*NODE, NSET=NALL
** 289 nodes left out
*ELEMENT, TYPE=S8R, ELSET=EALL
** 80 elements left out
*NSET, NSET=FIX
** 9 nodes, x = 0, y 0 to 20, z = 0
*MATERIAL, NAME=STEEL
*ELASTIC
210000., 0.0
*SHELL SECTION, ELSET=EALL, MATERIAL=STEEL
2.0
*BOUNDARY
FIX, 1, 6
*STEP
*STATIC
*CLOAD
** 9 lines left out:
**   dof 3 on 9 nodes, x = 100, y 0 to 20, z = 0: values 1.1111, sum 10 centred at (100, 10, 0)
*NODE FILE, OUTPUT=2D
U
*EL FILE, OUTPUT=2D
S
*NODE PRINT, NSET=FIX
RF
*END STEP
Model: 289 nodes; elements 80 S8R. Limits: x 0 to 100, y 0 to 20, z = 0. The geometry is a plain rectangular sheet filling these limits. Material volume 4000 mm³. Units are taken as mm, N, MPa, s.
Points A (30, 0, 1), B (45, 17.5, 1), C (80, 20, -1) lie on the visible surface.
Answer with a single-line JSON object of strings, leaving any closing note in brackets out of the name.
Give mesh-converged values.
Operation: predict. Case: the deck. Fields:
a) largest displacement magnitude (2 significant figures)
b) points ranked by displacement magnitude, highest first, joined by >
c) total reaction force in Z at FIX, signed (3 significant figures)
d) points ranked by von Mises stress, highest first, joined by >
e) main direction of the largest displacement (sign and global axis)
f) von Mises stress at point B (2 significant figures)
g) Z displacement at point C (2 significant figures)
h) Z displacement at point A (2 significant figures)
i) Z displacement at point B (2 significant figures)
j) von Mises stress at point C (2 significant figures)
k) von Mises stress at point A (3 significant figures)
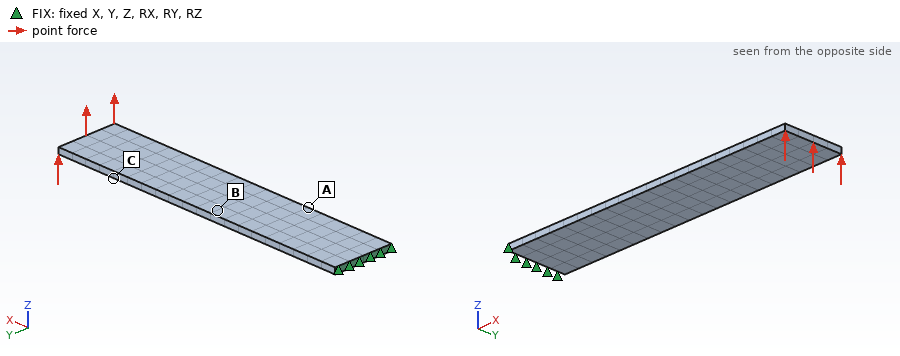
{"largest displacement magnitude": "1.2 mm", "points ranked by displacement magnitude, highest first, joined by >": "C > B > A", "total reaction force in Z at FIX, signed": "-10.0 N", "points ranked by von Mises stress, highest first, joined by >": "A > B > C", "main direction of the largest displacement": "+Z", "von Mises stress at point B": "41 MPa", "Z displacement at point C": "0.84 mm", "Z displacement at point A": "0.14 mm", "Z displacement at point B": "0.31 mm", "von Mises stress at point C": "15 MPa", "von Mises stress at point A": "52.5 MPa"}
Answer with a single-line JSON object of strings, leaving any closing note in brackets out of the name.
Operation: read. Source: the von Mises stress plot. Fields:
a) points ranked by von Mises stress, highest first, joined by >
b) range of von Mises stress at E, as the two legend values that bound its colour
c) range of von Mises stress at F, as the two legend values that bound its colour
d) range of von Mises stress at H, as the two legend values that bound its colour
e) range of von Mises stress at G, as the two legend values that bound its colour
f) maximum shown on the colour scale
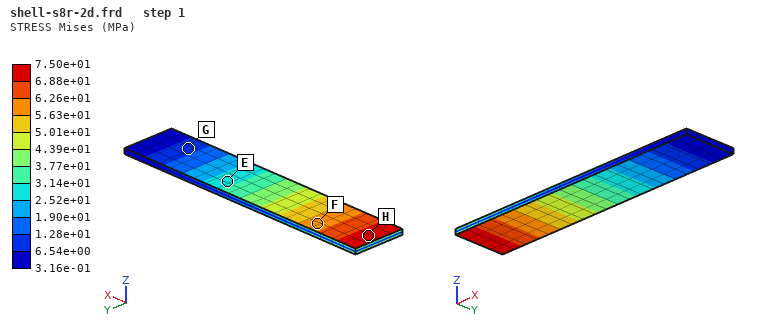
{"points ranked by von Mises stress, highest first, joined by >": "H > F > E > G", "range of von Mises stress at E, as the two legend values that bound its colour": "2.52e+01 to 3.14e+01 MPa", "range of von Mises stress at F, as the two legend values that bound its colour": "5.63e+01 to 6.26e+01 MPa", "range of von Mises stress at H, as the two legend values that bound its colour": "6.88e+01 to 7.50e+01 MPa", "range of von Mises stress at G, as the two legend values that bound its colour": "6.54e+00 to 1.28e+01 MPa", "maximum shown on the colour scale": "7.50e+01 MPa"}
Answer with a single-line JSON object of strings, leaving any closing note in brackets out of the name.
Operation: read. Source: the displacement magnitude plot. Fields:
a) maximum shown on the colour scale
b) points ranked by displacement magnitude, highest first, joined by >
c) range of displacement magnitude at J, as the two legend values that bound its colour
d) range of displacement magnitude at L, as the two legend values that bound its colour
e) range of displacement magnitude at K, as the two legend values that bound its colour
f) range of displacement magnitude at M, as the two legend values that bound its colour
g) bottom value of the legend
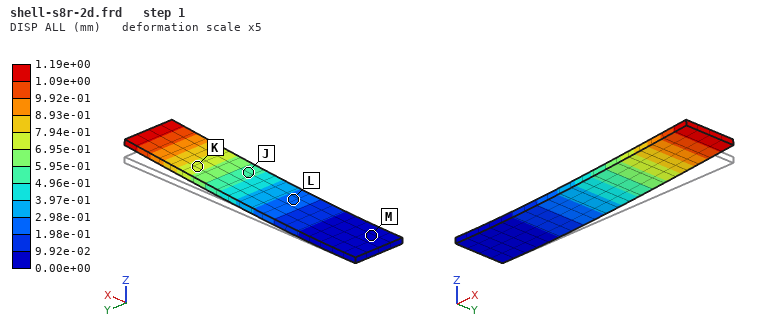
{"maximum shown on the colour scale": "1.19e+00 mm", "points ranked by displacement magnitude, highest first, joined by >": "K > J > L > M", "range of displacement magnitude at J, as the two legend values that bound its colour": "4.96e-01 to 5.95e-01 mm", "range of displacement magnitude at L, as the two legend values that bound its colour": "1.98e-01 to 2.98e-01 mm", "range of displacement magnitude at K, as the two legend values that bound its colour": "6.95e-01 to 7.94e-01 mm", "range of displacement magnitude at M, as the two legend values that bound its colour": "0.00e+00 to 9.92e-02 mm", "bottom value of the legend": "0.00e+00 mm"}
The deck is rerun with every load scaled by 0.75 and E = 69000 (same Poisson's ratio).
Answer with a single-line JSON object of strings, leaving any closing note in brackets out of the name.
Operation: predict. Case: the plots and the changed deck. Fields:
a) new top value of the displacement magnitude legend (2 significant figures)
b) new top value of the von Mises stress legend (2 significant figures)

{"new top value of the displacement magnitude legend": "2.7 mm", "new top value of the von Mises stress legend": "56 MPa"}
